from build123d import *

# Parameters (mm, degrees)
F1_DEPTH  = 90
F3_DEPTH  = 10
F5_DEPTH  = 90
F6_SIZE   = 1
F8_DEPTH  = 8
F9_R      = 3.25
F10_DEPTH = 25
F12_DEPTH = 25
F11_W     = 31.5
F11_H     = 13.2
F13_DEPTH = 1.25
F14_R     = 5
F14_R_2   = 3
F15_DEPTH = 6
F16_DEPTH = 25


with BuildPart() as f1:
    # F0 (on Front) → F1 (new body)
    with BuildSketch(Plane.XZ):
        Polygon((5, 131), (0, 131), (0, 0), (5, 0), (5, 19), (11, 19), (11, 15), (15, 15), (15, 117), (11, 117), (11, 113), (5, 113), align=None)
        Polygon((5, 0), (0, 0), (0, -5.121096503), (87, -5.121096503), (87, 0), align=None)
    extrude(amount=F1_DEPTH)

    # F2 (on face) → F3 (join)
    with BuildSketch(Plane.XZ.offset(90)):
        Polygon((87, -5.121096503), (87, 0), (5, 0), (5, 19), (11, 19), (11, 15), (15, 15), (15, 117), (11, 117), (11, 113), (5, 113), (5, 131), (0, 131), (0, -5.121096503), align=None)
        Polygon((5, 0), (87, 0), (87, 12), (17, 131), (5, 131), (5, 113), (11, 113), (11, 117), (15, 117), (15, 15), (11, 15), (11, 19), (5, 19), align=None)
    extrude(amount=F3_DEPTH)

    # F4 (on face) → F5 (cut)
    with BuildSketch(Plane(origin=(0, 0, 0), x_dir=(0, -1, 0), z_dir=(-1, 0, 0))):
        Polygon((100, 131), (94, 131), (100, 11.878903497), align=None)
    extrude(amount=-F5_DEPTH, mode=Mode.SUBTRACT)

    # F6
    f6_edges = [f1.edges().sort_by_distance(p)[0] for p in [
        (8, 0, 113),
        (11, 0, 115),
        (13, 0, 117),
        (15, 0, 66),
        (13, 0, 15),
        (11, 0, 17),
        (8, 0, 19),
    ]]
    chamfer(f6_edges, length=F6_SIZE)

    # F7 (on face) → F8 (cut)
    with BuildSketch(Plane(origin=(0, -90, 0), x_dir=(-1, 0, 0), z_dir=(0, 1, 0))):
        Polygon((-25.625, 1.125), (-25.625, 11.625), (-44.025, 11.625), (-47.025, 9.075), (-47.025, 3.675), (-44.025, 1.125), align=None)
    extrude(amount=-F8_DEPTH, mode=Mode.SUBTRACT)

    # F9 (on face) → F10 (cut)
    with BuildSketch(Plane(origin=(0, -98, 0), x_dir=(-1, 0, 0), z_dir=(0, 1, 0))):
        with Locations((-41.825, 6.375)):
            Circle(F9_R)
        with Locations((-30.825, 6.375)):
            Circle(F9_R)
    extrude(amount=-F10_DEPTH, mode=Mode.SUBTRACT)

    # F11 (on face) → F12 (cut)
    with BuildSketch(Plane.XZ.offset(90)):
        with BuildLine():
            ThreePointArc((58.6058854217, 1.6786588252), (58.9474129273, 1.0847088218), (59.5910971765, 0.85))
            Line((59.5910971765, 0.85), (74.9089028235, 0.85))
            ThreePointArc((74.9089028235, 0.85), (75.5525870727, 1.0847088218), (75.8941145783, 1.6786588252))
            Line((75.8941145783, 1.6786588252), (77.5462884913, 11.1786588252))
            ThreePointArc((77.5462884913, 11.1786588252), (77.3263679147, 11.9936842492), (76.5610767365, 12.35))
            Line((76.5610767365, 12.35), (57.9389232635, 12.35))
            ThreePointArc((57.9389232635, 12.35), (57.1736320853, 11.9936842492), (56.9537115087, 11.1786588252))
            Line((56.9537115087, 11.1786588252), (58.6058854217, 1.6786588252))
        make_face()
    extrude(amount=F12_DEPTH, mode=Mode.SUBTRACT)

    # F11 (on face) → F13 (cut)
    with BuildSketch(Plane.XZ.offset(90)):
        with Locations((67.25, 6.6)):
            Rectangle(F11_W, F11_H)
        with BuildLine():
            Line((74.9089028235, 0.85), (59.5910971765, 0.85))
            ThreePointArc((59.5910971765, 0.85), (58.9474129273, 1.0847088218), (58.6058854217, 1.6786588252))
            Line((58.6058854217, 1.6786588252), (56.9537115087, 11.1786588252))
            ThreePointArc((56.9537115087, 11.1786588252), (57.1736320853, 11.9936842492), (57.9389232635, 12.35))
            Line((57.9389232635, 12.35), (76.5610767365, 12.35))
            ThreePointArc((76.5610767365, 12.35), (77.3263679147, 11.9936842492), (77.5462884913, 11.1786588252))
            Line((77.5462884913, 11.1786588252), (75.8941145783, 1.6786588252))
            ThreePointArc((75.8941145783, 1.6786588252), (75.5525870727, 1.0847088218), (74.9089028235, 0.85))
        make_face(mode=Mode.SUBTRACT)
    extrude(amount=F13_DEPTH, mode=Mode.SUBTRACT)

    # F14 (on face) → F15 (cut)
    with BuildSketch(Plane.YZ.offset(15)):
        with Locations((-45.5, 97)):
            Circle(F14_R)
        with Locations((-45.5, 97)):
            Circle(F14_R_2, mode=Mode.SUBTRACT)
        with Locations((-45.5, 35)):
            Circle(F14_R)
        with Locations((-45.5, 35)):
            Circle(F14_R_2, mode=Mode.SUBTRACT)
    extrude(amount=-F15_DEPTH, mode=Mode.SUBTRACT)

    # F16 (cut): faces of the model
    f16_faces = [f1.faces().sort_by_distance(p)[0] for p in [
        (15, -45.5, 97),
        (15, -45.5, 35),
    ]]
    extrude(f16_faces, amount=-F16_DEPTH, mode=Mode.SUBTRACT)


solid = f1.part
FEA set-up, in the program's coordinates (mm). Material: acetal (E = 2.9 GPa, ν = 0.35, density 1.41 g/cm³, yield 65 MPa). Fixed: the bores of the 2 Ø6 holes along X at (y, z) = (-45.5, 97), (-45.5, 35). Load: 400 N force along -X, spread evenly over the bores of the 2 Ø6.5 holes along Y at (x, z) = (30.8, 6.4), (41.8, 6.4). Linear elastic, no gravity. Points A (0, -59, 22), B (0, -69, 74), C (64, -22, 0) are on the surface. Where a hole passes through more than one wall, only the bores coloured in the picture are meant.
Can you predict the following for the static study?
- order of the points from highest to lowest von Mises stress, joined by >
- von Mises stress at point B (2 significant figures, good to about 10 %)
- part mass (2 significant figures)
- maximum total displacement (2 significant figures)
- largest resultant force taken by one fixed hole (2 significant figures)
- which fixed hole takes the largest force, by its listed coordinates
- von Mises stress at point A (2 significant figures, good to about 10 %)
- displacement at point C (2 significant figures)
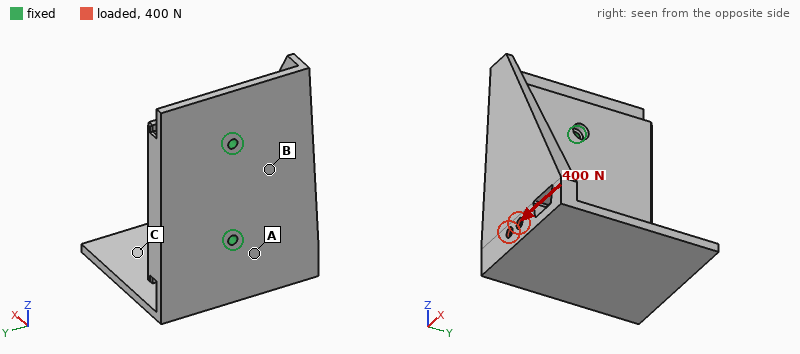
A > B > C
4.4 MPa
340 g
2.1 mm
560 N
(-45.5, 35)
6.0 MPa
1.2 mm
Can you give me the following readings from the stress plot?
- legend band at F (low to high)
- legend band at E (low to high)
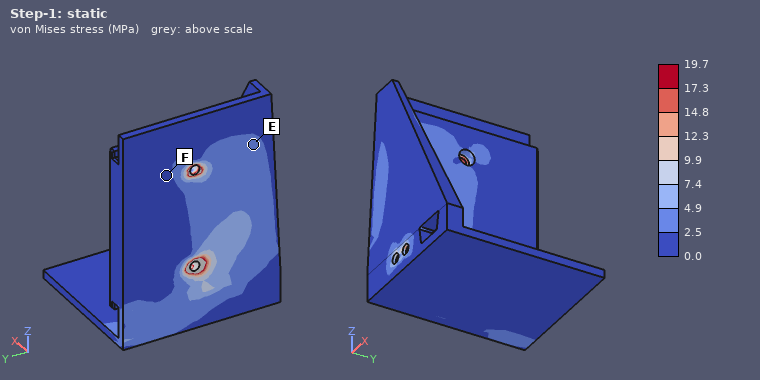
0.0 to 2.5 MPa
2.5 to 4.9 MPa
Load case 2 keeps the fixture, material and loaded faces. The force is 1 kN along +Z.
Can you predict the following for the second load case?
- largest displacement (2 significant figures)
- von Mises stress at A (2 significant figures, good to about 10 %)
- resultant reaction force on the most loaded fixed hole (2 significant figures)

1.00 mm
4.2 MPa
1.1 kN
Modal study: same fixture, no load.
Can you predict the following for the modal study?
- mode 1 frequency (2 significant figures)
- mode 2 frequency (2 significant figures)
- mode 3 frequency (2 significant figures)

240 Hz
250 Hz
550 Hz
